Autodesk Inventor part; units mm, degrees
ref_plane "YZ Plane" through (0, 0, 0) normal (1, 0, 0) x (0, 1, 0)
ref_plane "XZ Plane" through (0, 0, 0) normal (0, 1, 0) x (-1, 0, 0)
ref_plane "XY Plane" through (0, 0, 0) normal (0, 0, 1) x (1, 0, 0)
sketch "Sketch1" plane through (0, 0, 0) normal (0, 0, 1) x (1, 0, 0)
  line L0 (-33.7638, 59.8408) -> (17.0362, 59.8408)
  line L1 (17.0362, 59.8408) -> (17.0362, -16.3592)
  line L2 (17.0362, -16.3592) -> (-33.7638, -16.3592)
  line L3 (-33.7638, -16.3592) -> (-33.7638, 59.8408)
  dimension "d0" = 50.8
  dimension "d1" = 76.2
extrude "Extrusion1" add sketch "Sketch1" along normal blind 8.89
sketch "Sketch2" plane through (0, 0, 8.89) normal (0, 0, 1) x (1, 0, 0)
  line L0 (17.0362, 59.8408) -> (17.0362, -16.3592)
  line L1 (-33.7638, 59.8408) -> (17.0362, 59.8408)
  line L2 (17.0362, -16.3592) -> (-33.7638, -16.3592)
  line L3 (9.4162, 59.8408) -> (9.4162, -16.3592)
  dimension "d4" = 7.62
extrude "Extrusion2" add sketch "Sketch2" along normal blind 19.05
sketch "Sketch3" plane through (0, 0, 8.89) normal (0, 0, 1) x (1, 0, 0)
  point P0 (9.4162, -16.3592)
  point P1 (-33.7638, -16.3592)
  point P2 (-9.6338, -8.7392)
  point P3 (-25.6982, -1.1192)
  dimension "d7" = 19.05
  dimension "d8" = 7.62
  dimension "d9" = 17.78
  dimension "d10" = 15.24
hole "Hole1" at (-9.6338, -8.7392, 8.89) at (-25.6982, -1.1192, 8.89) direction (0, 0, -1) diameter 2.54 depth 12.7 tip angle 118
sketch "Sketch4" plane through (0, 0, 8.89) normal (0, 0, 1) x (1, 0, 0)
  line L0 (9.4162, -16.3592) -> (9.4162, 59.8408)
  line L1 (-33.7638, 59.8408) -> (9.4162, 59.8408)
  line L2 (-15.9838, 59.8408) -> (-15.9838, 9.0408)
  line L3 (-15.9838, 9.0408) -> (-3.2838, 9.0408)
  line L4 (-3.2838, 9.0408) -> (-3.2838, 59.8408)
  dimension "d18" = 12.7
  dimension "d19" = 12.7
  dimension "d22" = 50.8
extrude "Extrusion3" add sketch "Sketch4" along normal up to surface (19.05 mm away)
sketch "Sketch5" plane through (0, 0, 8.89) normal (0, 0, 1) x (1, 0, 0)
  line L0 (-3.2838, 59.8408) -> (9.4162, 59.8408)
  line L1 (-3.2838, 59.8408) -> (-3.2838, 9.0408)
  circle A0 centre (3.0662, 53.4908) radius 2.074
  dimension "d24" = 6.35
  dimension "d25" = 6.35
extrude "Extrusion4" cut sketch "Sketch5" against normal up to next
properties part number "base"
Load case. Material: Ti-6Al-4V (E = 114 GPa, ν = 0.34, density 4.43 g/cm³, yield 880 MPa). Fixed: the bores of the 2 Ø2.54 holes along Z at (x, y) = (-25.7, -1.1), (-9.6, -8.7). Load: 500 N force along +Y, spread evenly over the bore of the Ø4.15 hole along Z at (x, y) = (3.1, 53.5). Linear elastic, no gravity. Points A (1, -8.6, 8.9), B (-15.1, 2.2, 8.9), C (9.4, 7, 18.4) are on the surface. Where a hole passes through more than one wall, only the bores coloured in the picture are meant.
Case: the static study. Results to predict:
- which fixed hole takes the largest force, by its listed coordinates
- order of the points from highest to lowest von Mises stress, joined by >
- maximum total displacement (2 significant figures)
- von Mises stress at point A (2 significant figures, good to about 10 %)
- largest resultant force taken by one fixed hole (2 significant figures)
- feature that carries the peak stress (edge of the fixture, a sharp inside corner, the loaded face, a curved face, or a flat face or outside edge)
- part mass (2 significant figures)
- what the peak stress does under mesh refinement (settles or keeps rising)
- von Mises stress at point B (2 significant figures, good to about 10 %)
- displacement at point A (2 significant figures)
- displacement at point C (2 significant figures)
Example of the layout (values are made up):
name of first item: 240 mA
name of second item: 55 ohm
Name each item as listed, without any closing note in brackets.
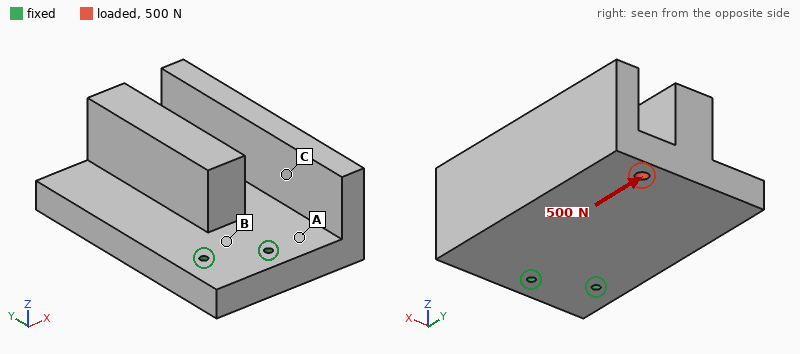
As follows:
which fixed hole takes the largest force, by its listed coordinates: (-9.6, -8.7)
order of the points from highest to lowest von Mises stress, joined by >: B > A > C
maximum total displacement: 5.8 µm
von Mises stress at point A: 2.1 MPa
largest resultant force taken by one fixed hole: 770 N
feature that carries the peak stress: edge of the fixture
part mass: 250 g
what the peak stress does under mesh refinement: keeps rising
von Mises stress at point B: 3.4 MPa
displacement at point A: 1.3 µm
displacement at point C: 2.4 µm
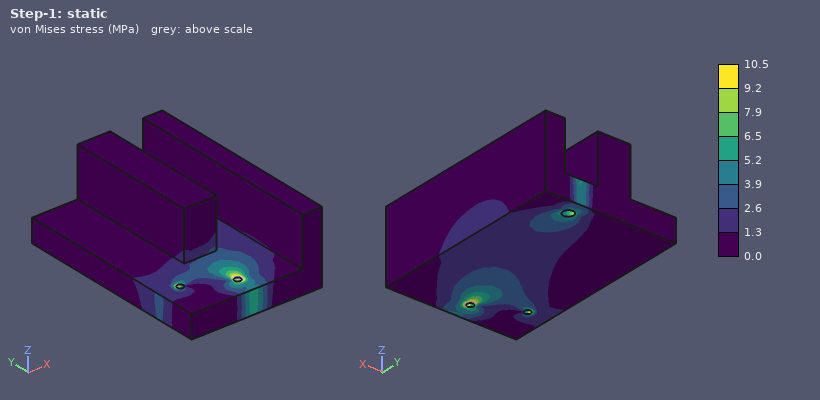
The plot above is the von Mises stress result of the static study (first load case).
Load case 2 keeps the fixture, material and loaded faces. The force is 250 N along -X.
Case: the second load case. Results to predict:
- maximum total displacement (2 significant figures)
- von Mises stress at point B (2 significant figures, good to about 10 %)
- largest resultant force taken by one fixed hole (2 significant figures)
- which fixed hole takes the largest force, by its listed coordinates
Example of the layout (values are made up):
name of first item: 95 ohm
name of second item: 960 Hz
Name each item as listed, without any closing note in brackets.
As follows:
maximum total displacement: 8.1 µm
von Mises stress at point B: 4.3 MPa
largest resultant force taken by one fixed hole: 820 N
which fixed hole takes the largest force, by its listed coordinates: (-25.7, -1.1)
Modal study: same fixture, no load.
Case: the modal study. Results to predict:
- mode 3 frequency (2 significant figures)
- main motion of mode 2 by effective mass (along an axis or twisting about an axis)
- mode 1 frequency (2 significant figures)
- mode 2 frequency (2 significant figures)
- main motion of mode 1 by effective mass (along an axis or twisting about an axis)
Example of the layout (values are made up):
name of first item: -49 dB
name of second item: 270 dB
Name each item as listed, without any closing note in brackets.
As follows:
mode 3 frequency: 3400 Hz
main motion of mode 2 by effective mass: along X
mode 1 frequency: 1100 Hz
mode 2 frequency: 2600 Hz
main motion of mode 1 by effective mass: along Z
